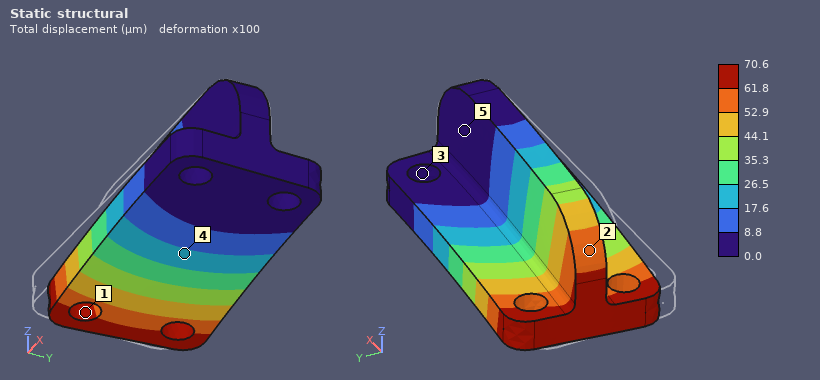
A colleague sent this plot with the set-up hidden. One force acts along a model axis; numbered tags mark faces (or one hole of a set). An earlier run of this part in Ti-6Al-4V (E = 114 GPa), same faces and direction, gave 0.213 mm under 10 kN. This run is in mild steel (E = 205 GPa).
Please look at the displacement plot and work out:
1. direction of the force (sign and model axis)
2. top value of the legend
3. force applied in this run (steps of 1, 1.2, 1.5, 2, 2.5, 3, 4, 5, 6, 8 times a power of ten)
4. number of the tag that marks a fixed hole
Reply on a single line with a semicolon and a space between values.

+Y; 70.6 µm; 6 kN; 3
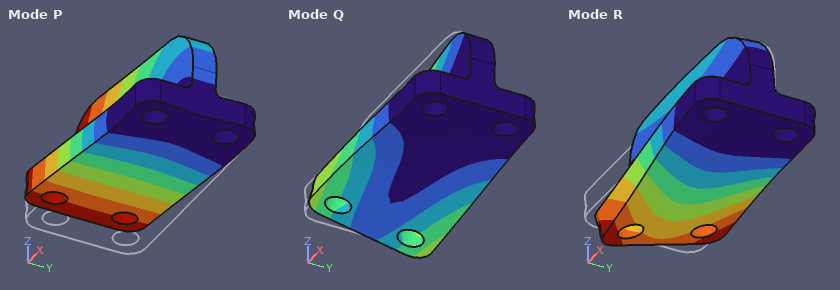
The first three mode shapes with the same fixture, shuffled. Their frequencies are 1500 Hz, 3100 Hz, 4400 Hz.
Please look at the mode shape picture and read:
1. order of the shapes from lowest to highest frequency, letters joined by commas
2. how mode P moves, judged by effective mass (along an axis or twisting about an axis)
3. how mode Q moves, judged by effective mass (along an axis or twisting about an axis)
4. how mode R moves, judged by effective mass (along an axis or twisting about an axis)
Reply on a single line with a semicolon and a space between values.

P, Q, R; along Z; along Y; along Y
